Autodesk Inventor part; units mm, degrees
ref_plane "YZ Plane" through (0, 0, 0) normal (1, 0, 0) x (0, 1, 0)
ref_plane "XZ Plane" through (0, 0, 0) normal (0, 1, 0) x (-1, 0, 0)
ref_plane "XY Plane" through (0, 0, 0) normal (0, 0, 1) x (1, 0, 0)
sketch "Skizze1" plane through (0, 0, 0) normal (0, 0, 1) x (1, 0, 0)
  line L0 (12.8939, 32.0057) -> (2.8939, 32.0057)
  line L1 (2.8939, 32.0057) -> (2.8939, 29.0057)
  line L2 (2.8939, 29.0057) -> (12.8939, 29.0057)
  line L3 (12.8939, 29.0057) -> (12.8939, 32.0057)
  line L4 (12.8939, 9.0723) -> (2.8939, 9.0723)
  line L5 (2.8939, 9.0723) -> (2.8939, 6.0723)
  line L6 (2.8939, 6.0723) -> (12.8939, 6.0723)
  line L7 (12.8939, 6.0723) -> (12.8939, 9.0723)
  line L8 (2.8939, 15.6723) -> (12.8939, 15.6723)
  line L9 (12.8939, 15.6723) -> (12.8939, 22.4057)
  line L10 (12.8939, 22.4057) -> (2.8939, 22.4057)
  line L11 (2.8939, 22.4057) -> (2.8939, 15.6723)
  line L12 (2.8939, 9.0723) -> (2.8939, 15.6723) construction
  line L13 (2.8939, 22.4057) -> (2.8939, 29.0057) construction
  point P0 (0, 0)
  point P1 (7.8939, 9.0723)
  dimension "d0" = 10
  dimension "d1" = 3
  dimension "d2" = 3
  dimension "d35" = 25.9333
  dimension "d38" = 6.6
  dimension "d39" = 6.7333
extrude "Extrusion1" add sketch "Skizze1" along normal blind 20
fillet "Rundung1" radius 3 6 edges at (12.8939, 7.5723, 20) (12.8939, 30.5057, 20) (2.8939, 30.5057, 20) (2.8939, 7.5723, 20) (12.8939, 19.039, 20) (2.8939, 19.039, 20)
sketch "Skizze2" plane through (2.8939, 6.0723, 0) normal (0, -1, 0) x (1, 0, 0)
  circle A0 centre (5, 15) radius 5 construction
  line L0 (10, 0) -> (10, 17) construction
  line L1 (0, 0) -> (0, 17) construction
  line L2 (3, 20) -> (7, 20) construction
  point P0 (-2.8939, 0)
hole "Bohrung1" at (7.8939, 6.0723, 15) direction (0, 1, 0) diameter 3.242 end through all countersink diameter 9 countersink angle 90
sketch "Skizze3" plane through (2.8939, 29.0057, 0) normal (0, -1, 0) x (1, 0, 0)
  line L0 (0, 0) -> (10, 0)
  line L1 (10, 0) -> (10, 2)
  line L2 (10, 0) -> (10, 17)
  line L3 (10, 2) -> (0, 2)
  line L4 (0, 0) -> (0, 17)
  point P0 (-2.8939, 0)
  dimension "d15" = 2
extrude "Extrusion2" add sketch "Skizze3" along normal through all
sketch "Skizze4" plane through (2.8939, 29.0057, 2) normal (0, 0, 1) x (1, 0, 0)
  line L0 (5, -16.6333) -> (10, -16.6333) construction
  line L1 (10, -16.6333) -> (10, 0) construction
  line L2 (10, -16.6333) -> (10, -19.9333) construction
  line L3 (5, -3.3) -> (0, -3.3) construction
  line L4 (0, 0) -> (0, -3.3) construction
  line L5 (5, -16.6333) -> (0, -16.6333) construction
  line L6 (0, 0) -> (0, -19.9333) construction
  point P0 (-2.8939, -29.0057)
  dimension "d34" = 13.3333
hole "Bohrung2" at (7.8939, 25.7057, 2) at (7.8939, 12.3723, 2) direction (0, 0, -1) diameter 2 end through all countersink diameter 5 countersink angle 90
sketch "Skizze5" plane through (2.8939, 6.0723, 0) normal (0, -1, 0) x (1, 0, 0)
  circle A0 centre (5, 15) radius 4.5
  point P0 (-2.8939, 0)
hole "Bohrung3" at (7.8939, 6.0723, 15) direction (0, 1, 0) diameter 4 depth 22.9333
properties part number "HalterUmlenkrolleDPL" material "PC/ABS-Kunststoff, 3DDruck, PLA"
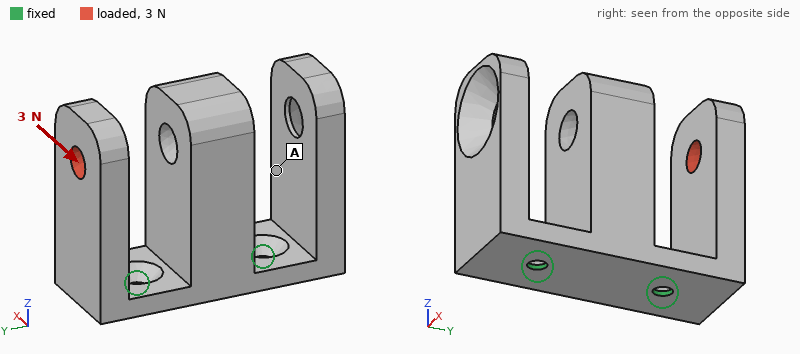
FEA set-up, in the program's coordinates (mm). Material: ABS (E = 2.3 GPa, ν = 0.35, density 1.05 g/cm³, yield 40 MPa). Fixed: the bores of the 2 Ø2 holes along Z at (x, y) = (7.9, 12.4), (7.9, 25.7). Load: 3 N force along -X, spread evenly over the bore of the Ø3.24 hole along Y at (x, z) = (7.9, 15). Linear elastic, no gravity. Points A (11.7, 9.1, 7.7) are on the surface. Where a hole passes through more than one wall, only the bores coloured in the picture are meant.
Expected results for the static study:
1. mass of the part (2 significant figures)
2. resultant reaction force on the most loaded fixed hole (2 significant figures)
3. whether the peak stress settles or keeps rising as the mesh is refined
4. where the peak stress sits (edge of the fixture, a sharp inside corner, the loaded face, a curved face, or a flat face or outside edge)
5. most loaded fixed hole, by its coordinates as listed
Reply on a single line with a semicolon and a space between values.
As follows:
2.7 g; 3.4 N; keeps rising; edge of the fixture; (7.9, 25.7)
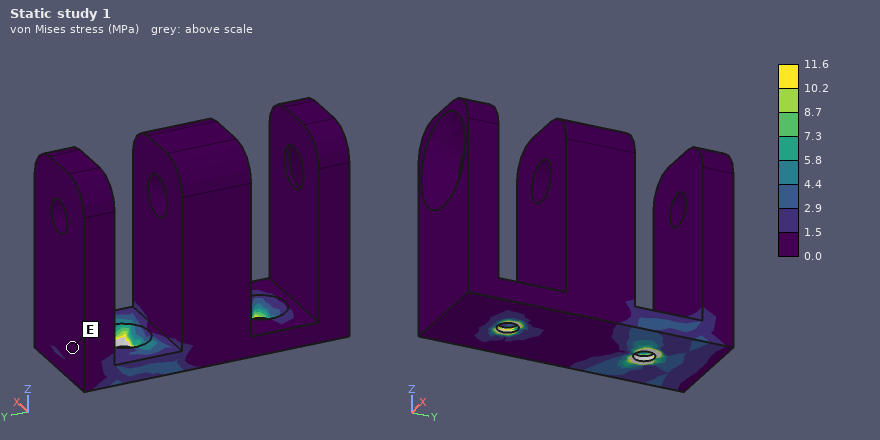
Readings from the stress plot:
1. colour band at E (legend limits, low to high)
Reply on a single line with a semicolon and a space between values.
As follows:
0.0 to 1.5 MPa
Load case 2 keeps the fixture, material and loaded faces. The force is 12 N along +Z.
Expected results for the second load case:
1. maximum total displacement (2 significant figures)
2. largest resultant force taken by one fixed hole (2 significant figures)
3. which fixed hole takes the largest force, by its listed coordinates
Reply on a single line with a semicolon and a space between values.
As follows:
0.35 mm; 18 N; (7.9, 25.7)
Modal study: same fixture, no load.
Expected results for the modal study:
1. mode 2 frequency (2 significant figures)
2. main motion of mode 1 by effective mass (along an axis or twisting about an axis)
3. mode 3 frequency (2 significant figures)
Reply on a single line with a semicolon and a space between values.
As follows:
840 Hz; along X; 960 Hz
